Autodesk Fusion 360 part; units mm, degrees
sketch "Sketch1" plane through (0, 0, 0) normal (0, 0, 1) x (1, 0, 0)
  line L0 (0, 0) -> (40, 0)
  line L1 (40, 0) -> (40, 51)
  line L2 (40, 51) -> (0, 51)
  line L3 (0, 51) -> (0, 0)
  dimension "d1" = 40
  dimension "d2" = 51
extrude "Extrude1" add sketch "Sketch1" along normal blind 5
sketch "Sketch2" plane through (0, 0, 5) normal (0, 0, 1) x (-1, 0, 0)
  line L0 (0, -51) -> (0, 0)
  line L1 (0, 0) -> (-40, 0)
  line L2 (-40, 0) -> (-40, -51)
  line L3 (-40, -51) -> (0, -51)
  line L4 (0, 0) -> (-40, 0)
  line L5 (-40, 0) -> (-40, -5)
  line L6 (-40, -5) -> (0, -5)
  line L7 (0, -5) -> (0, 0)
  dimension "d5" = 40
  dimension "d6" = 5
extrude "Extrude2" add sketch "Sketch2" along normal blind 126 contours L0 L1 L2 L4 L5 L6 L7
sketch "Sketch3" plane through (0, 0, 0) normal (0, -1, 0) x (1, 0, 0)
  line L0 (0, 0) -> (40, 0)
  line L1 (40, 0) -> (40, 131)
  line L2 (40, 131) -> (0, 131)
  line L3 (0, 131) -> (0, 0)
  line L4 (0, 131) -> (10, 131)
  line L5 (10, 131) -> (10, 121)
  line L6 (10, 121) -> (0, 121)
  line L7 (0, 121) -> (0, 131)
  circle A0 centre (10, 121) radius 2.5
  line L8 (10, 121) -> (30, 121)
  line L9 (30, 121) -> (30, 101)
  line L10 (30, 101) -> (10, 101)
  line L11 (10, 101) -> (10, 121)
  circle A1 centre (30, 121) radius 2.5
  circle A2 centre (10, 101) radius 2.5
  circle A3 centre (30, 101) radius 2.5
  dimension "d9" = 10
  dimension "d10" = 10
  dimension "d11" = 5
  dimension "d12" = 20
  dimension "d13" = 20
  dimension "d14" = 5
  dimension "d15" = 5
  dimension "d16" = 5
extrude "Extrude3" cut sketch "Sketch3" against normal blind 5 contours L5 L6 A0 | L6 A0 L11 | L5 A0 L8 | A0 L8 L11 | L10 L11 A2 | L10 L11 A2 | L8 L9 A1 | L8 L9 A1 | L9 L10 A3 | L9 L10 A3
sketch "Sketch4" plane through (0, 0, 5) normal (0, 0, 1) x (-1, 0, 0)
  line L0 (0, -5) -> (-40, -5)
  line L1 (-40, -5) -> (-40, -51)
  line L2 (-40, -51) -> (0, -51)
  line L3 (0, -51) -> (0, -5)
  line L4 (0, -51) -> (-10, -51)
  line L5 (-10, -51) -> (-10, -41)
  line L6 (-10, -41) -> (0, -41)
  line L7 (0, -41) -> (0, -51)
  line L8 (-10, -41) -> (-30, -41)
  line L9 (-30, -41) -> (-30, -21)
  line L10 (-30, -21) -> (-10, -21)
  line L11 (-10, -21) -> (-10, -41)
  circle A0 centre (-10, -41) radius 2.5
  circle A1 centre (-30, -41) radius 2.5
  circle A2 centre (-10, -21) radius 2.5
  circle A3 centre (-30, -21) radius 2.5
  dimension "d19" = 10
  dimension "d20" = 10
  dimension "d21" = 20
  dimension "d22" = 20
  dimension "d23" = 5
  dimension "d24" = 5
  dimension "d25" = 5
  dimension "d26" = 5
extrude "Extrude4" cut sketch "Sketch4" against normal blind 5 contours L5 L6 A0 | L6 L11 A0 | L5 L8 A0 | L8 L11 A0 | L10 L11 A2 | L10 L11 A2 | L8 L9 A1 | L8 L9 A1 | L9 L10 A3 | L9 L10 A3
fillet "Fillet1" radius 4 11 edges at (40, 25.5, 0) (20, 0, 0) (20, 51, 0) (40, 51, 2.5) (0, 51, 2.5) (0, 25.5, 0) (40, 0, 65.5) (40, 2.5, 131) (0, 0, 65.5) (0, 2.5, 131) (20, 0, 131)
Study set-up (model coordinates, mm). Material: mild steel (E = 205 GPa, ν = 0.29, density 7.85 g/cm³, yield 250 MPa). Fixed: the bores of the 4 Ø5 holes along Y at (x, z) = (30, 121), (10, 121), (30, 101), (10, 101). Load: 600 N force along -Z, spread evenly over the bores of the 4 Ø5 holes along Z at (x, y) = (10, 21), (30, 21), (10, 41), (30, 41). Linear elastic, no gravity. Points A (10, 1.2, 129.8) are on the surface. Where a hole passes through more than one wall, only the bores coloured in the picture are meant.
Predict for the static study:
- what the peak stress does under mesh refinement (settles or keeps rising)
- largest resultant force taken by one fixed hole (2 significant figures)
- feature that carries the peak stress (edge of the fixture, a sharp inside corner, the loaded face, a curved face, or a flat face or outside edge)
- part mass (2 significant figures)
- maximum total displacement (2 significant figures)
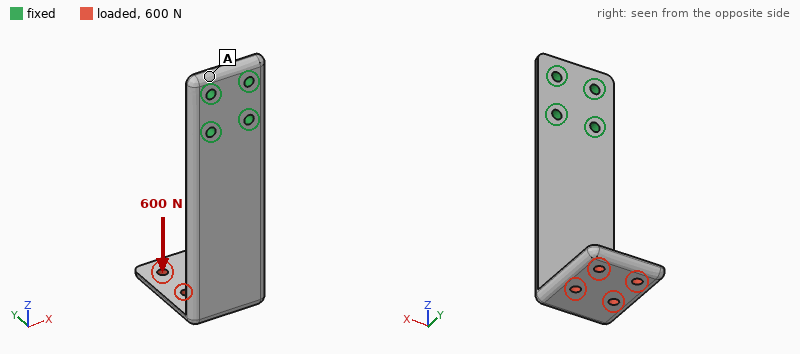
keeps rising
240 N
edge of the fixture
260 g
1.5 mm
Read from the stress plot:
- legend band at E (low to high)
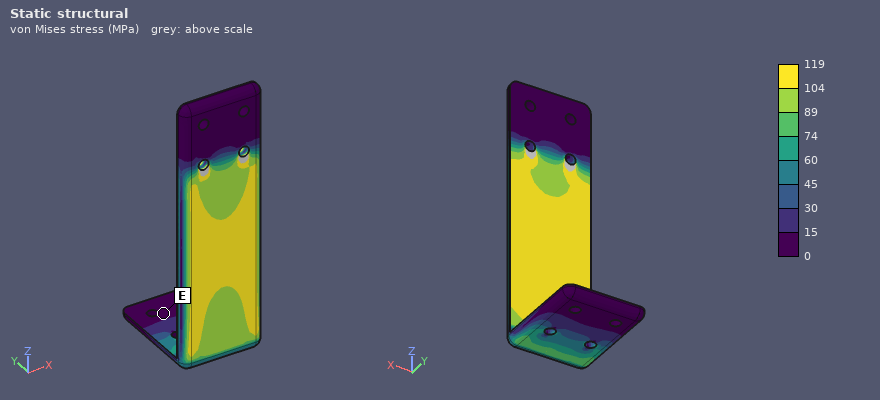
0 to 15 MPa
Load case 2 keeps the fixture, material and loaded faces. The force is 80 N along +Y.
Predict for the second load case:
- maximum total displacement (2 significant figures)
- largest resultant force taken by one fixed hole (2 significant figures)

0.38 mm
77 N
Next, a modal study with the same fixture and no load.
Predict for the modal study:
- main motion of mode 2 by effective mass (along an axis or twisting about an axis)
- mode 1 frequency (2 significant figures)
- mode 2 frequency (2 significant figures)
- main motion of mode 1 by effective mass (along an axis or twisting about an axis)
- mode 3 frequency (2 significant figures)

along X
240 Hz
700 Hz
along Y
1000 Hz
